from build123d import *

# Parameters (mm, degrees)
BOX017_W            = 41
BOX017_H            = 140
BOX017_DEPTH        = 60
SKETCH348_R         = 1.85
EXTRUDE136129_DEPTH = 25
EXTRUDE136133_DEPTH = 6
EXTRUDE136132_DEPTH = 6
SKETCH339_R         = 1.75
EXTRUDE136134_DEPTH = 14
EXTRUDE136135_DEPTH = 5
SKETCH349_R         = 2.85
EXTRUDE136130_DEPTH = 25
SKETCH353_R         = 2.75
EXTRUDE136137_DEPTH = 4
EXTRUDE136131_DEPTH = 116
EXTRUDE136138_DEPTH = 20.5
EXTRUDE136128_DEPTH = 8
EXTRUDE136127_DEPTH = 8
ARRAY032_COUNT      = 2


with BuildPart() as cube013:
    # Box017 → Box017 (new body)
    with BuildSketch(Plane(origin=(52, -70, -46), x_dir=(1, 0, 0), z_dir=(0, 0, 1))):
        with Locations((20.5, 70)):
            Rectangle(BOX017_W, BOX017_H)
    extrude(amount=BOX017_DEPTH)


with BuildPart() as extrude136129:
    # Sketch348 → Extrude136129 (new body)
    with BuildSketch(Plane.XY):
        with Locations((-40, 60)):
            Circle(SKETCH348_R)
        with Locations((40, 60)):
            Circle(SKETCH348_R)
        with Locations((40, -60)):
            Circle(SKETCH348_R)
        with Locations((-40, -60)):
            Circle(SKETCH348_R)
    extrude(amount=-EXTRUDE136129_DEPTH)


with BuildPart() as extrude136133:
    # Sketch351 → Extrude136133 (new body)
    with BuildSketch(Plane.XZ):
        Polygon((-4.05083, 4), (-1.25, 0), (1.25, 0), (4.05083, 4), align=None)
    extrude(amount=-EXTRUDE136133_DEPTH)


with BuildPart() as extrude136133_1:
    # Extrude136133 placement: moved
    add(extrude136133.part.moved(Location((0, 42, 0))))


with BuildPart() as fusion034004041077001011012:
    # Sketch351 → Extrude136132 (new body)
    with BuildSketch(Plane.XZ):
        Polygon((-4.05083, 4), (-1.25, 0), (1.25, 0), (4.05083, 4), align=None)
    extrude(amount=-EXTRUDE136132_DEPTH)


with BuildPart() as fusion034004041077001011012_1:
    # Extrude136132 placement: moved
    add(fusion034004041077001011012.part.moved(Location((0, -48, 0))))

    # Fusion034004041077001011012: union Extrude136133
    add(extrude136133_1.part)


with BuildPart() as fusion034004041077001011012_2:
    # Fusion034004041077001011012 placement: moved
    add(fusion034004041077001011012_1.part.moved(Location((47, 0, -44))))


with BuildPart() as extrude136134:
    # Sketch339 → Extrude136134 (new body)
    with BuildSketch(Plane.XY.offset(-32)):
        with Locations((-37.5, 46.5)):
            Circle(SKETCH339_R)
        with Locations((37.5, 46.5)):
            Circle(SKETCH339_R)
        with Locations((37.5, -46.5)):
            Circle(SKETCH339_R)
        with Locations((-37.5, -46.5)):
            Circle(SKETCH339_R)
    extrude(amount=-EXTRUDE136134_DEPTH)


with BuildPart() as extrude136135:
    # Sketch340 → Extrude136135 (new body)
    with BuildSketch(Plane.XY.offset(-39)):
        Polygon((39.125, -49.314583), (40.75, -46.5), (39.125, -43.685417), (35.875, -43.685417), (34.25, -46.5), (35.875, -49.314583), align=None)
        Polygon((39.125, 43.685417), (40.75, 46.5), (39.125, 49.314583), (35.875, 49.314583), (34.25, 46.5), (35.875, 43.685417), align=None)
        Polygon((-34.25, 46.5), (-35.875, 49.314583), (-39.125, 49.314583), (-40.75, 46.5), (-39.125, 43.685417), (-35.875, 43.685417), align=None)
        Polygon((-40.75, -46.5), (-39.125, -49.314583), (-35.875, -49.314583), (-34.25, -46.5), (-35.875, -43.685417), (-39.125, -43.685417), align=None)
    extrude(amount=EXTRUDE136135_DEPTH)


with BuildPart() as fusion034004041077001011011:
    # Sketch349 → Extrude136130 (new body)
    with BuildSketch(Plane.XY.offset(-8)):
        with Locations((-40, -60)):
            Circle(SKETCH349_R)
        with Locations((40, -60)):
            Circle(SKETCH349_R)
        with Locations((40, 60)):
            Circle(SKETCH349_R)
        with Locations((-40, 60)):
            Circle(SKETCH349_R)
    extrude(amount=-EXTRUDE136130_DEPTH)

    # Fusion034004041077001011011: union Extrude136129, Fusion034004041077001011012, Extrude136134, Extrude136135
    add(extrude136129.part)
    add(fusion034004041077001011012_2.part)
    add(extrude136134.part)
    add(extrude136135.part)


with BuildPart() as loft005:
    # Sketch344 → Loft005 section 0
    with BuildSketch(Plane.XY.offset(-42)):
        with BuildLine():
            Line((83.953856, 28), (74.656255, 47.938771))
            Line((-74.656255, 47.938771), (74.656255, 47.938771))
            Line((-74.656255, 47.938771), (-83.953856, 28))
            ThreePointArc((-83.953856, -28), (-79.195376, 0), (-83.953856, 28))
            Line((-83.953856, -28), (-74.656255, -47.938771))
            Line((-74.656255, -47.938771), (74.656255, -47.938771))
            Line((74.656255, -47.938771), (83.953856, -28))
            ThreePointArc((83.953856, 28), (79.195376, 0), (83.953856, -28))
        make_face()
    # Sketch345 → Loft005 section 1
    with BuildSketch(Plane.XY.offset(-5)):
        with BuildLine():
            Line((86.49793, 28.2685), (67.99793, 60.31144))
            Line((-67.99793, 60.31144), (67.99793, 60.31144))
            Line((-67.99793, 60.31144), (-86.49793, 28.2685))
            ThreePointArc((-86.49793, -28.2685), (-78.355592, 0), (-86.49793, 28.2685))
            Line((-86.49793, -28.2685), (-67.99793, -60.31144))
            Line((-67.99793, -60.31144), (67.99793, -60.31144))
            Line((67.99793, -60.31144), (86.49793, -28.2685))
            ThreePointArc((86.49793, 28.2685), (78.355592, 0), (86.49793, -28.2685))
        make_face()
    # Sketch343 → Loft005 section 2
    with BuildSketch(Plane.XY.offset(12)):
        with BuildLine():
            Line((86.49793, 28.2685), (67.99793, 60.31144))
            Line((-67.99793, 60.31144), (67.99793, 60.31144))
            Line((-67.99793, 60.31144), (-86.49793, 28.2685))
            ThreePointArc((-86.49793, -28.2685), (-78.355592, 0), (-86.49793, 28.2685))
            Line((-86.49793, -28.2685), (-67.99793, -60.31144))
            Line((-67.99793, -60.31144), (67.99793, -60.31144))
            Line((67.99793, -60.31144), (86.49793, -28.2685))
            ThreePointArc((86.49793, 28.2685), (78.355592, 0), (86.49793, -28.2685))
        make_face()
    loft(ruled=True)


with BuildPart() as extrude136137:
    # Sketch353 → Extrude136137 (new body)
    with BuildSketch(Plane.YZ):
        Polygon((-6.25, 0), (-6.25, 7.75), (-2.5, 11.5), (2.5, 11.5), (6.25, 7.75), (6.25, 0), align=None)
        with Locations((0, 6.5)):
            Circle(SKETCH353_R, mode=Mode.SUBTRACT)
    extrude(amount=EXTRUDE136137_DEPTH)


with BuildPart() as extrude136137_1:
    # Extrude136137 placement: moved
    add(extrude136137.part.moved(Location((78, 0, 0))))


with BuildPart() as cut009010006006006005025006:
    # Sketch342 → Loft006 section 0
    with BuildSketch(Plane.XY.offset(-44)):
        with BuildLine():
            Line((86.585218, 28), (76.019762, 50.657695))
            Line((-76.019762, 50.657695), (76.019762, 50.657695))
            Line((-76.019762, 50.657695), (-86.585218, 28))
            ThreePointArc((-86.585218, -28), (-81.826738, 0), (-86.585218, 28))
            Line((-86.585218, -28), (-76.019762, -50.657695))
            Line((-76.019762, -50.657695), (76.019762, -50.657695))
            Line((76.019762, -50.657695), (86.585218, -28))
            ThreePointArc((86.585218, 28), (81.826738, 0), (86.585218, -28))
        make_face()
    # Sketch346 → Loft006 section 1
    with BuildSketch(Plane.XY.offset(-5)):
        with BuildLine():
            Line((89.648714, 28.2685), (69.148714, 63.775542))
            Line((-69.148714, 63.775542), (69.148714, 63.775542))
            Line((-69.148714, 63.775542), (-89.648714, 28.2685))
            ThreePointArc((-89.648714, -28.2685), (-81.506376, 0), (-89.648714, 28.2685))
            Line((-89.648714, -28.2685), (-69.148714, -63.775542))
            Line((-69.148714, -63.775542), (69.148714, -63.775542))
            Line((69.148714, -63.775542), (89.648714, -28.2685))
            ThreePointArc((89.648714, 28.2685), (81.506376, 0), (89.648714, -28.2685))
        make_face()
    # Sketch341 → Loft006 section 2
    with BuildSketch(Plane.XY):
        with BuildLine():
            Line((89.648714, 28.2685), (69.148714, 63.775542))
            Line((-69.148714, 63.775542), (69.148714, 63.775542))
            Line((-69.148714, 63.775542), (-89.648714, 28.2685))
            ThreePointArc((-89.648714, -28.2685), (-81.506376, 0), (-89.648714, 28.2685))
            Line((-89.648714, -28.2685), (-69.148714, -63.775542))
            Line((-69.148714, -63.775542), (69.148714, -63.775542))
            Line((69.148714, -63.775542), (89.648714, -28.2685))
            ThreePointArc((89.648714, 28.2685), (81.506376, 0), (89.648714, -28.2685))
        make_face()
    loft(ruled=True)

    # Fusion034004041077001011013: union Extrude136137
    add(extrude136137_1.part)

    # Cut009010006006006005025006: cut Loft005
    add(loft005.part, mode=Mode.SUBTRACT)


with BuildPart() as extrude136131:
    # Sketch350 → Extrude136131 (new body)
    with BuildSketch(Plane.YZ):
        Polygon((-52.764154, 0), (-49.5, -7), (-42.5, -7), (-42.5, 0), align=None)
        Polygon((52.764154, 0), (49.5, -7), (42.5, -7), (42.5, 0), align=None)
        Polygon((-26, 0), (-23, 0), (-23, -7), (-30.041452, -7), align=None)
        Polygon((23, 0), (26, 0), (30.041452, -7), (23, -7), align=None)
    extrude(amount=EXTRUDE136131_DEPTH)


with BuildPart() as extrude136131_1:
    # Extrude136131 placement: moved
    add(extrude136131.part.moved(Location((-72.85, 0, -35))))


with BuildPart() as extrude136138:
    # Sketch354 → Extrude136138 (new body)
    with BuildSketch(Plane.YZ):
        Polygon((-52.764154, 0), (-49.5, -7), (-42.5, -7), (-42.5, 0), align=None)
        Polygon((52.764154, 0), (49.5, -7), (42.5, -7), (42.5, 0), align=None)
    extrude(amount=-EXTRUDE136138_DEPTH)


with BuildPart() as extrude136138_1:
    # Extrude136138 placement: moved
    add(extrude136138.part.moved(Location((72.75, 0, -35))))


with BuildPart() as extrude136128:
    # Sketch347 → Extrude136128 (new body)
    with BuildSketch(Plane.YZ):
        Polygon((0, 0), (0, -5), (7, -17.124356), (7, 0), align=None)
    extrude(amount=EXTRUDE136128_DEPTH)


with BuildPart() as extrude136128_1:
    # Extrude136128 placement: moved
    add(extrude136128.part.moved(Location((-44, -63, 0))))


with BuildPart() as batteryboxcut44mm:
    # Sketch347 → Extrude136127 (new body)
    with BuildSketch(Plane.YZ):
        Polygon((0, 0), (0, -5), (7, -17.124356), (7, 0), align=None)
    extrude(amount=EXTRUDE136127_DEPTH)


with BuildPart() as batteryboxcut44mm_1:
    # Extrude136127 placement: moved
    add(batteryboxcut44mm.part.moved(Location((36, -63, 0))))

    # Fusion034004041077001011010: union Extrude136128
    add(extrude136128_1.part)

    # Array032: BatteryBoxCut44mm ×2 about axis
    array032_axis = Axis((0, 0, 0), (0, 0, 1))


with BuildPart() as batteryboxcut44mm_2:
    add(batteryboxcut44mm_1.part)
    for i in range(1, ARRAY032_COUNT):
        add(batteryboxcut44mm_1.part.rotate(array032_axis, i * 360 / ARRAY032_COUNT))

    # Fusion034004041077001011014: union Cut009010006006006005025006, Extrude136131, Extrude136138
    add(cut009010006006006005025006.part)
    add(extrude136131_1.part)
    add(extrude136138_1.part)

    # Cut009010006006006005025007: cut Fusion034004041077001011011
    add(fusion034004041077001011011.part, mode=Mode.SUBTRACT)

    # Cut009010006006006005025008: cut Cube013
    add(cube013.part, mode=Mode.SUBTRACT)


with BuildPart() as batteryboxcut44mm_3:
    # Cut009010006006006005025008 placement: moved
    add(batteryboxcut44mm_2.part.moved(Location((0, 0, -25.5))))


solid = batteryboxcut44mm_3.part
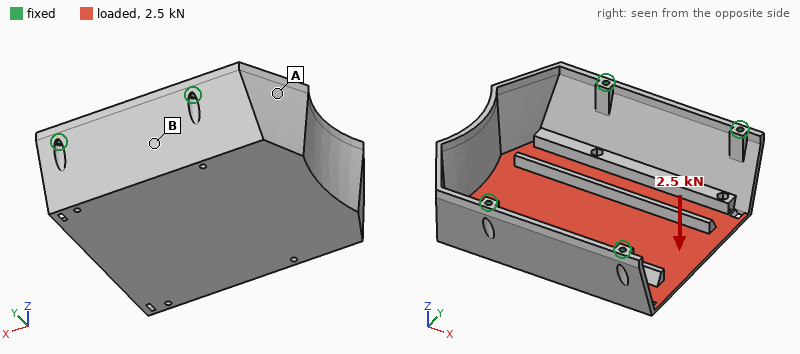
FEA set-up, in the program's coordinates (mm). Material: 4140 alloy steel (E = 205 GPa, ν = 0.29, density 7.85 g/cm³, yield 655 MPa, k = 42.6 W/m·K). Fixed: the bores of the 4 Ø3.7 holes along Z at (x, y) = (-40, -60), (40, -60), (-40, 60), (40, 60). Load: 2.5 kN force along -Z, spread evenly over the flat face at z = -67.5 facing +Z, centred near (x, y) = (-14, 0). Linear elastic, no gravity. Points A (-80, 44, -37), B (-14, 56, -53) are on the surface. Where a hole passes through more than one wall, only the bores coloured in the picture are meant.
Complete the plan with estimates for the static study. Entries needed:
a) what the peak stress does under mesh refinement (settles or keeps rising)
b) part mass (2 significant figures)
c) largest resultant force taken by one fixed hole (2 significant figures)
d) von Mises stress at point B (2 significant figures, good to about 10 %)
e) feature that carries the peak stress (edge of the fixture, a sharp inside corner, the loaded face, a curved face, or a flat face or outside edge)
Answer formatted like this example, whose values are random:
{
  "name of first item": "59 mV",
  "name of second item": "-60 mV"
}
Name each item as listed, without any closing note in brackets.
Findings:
{
  "what the peak stress does under mesh refinement": "keeps rising",
  "part mass": "750 g",
  "largest resultant force taken by one fixed hole": "1.0 kN",
  "von Mises stress at point B": "28 MPa",
  "feature that carries the peak stress": "a sharp inside corner"
}
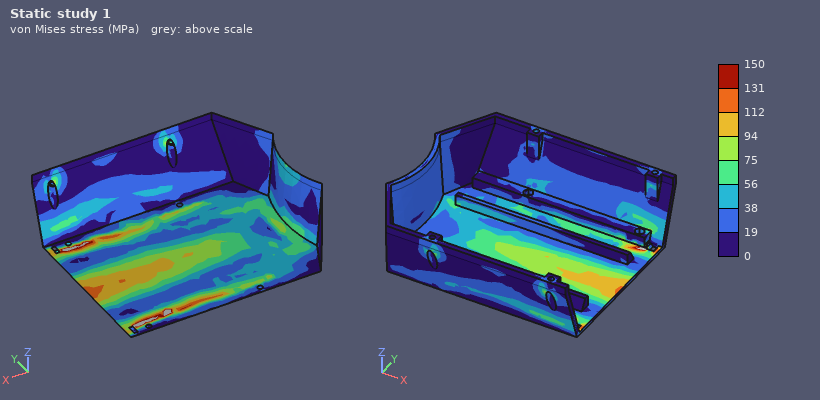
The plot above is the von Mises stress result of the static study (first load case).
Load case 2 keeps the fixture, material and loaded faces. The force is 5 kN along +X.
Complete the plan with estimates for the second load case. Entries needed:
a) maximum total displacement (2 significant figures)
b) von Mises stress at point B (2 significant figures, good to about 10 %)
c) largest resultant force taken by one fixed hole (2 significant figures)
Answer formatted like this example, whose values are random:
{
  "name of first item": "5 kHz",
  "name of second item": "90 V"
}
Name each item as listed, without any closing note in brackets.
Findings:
{
  "maximum total displacement": "16 µm",
  "von Mises stress at point B": "19 MPa",
  "largest resultant force taken by one fixed hole": "1.7 kN"
}
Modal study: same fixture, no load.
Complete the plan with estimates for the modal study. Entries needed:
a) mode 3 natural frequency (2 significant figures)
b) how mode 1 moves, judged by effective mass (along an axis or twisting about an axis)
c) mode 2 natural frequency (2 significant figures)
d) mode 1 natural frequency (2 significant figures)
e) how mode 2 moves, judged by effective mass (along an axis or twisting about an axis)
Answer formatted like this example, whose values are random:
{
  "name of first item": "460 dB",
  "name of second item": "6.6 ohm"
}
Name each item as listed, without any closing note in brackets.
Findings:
{
  "mode 3 natural frequency": "1700 Hz",
  "how mode 1 moves, judged by effective mass": "along Y",
  "mode 2 natural frequency": "1300 Hz",
  "mode 1 natural frequency": "960 Hz",
  "how mode 2 moves, judged by effective mass": "along Z"
}
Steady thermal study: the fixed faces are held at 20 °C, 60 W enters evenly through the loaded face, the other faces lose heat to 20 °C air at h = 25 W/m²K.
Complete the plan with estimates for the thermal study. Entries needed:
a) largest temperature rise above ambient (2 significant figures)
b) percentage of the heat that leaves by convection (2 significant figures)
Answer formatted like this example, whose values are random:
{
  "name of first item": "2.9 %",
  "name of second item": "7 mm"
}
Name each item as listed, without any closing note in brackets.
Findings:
{
  "largest temperature rise above ambient": "72 K",
  "percentage of the heat that leaves by convection": "72 %"
}
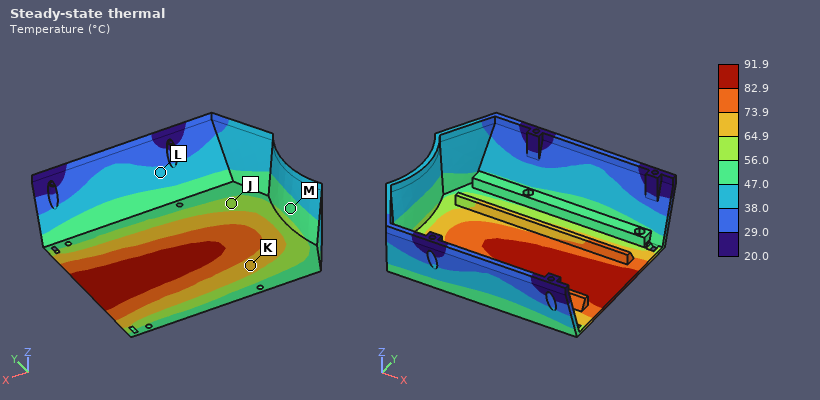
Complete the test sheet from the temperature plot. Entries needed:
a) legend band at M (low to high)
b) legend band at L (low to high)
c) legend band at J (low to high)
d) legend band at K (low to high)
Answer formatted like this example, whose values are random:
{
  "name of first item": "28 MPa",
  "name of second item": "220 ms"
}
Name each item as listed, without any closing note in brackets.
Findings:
{
  "legend band at M": "47.0 to 56.0 °C",
  "legend band at L": "38.0 to 47.0 °C",
  "legend band at J": "56.0 to 64.9 °C",
  "legend band at K": "64.9 to 73.9 °C"
}
